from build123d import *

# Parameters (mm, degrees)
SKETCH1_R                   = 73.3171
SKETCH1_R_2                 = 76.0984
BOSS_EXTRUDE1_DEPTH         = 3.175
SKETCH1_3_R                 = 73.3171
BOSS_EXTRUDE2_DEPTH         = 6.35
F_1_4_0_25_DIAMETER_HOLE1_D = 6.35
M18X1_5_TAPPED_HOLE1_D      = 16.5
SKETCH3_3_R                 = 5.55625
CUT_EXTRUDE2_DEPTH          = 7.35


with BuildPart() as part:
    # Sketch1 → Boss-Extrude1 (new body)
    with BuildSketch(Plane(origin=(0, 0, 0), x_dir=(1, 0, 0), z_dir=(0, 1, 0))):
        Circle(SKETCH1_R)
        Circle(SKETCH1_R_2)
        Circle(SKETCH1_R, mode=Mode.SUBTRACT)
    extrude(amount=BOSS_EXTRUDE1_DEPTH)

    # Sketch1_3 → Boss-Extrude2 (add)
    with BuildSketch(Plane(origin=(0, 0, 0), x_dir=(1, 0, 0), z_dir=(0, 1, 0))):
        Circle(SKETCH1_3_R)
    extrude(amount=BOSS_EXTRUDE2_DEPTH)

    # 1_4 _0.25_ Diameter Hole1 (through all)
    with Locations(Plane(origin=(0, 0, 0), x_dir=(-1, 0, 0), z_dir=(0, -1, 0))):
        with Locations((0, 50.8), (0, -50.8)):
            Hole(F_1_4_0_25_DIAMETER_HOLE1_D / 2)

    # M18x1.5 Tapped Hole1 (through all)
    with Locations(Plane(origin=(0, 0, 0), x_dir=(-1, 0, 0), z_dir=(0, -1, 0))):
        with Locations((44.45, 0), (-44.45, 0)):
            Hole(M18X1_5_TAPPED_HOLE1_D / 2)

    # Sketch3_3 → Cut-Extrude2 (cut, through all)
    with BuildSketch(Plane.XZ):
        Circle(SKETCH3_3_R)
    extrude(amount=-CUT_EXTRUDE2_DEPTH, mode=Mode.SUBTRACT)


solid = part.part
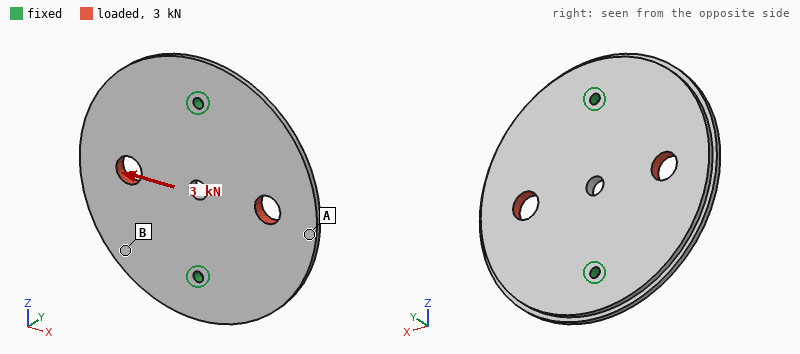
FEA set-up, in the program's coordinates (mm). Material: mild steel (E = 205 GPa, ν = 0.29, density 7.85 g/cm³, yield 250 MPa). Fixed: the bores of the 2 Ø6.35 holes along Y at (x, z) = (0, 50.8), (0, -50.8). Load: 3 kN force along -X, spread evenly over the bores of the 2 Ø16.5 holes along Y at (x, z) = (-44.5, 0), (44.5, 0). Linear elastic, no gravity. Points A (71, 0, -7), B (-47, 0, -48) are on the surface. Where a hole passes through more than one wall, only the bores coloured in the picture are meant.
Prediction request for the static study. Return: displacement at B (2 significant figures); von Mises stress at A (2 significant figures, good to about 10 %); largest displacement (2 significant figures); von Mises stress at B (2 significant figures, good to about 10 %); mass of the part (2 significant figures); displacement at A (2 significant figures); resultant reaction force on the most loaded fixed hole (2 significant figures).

0.80 µm
3.9 MPa
2.1 µm
1.6 MPa
850 g
1.8 µm
1.5 kN
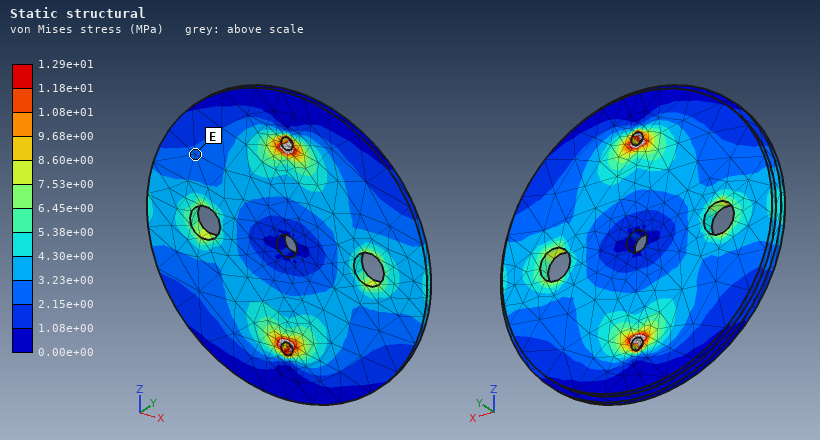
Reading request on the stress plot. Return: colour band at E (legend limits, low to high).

2.15e+00 to 3.23e+00 MPa
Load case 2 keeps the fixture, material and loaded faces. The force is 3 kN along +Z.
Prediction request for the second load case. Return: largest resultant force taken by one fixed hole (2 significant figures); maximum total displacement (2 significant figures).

1.5 kN
2.2 µm
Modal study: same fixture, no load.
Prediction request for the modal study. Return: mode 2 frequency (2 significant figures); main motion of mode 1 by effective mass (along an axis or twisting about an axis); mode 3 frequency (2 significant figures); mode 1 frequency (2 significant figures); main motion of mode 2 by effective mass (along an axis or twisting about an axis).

1100 Hz
twisting about Z
2200 Hz
860 Hz
along Y
